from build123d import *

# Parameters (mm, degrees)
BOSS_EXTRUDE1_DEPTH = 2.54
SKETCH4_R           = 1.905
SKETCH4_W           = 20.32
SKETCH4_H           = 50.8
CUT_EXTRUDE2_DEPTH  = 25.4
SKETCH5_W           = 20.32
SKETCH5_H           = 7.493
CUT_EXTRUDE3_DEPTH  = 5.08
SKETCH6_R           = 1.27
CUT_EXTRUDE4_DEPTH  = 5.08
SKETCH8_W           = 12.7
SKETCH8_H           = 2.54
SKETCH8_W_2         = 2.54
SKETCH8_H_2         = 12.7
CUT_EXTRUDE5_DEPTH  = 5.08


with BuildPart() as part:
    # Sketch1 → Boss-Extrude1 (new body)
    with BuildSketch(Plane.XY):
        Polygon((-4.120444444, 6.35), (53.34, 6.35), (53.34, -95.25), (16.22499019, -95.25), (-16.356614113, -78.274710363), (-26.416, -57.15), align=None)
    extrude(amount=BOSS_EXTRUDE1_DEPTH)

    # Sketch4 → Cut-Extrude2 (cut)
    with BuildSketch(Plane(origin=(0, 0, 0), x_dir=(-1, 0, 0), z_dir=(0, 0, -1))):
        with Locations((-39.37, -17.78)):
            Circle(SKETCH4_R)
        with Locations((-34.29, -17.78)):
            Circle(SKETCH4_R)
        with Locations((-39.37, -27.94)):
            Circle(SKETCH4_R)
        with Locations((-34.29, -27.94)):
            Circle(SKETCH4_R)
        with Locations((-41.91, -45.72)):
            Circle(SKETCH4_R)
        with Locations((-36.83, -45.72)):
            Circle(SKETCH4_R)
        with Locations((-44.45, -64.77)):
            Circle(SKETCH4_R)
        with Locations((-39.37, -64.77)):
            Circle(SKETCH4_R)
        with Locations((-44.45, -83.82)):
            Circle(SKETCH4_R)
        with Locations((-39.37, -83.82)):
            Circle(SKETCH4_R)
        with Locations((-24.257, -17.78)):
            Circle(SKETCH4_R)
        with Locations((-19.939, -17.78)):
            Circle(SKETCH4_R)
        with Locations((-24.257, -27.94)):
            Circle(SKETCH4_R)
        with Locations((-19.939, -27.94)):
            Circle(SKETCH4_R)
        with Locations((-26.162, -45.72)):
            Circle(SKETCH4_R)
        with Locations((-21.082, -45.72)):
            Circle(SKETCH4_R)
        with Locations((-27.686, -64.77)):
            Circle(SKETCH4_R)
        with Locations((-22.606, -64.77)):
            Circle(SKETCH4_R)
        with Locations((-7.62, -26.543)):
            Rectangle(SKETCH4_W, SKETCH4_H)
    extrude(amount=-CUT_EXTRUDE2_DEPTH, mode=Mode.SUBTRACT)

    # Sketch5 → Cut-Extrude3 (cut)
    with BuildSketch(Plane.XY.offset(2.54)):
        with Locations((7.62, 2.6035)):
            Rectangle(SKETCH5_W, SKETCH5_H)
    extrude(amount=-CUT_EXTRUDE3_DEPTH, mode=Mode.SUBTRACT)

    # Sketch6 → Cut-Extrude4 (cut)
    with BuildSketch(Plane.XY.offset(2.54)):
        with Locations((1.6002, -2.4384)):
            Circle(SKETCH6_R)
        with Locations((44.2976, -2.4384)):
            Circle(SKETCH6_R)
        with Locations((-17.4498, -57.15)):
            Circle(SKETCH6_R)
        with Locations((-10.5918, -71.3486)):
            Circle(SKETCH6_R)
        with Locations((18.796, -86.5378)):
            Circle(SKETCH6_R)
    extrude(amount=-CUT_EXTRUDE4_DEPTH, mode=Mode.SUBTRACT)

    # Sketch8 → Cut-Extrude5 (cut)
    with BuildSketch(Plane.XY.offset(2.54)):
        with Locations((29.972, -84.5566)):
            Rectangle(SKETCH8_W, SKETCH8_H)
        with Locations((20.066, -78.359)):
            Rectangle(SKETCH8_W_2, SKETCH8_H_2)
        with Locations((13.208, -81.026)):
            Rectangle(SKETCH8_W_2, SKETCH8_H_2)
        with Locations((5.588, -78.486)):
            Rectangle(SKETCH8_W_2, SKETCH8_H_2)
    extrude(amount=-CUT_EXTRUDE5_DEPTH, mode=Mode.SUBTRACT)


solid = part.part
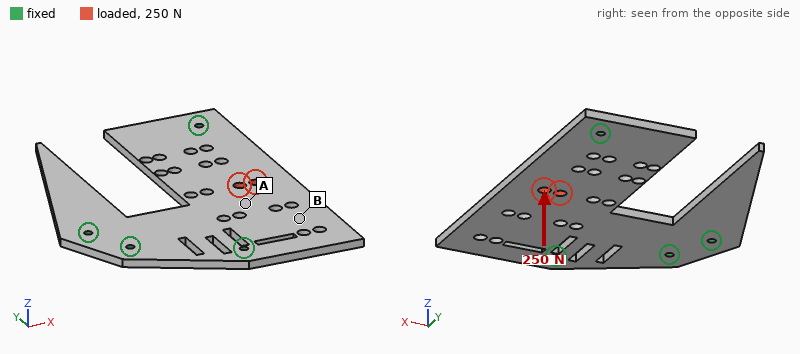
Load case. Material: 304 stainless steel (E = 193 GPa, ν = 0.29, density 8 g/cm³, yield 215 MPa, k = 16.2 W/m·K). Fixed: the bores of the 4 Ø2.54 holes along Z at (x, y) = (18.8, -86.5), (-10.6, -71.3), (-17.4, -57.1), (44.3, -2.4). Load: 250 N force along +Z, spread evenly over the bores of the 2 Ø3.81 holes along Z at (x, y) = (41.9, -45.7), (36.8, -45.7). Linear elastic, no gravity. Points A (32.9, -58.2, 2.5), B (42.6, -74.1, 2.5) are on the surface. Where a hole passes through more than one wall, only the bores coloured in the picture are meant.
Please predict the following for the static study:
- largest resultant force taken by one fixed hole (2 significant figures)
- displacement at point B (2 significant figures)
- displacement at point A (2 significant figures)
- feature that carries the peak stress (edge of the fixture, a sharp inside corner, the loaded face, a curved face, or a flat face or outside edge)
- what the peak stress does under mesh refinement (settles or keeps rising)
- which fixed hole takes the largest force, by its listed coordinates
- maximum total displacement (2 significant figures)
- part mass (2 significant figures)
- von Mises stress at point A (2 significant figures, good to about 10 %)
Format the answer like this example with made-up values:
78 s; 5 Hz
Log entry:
120 N; 0.11 mm; 0.12 mm; edge of the fixture; keeps rising; (44.3, -2.4); 0.21 mm; 110 g; 30 MPa
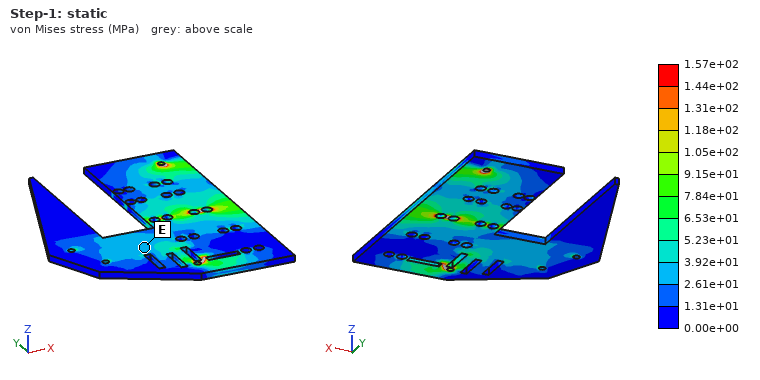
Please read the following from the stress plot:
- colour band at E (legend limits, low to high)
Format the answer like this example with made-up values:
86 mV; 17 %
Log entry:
2.61e+01 to 3.92e+01 MPa
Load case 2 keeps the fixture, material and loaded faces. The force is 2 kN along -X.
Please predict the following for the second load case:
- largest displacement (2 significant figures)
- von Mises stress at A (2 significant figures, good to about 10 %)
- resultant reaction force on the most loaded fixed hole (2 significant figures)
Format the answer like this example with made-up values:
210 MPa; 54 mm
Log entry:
15 µm; 29 MPa; 750 N
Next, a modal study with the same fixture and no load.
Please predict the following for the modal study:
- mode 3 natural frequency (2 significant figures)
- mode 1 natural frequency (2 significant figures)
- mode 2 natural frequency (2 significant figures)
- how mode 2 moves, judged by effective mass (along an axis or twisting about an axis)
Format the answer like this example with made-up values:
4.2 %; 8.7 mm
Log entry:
2000 Hz; 860 Hz; 1200 Hz; along Z
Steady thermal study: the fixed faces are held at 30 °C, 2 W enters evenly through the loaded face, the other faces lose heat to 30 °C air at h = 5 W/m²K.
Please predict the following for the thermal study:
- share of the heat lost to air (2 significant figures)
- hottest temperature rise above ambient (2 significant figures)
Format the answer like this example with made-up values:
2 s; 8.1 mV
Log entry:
32 %; 40 K
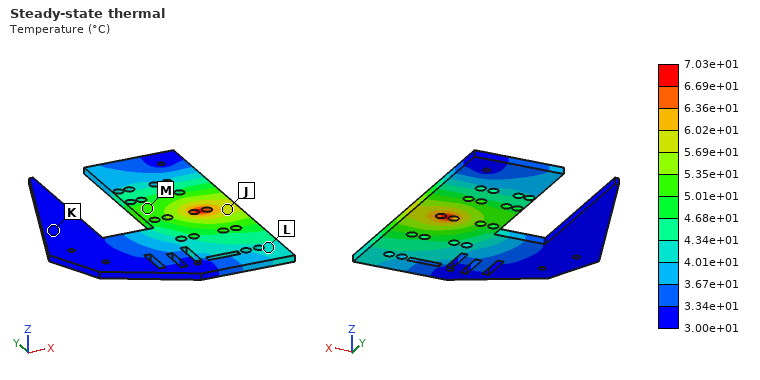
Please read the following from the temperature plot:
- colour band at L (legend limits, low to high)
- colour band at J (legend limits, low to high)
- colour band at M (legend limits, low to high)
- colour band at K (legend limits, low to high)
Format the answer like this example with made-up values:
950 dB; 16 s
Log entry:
4.01e+01 to 4.34e+01 °C; 5.69e+01 to 6.02e+01 °C; 5.01e+01 to 5.35e+01 °C; 3.00e+01 to 3.34e+01 °C
